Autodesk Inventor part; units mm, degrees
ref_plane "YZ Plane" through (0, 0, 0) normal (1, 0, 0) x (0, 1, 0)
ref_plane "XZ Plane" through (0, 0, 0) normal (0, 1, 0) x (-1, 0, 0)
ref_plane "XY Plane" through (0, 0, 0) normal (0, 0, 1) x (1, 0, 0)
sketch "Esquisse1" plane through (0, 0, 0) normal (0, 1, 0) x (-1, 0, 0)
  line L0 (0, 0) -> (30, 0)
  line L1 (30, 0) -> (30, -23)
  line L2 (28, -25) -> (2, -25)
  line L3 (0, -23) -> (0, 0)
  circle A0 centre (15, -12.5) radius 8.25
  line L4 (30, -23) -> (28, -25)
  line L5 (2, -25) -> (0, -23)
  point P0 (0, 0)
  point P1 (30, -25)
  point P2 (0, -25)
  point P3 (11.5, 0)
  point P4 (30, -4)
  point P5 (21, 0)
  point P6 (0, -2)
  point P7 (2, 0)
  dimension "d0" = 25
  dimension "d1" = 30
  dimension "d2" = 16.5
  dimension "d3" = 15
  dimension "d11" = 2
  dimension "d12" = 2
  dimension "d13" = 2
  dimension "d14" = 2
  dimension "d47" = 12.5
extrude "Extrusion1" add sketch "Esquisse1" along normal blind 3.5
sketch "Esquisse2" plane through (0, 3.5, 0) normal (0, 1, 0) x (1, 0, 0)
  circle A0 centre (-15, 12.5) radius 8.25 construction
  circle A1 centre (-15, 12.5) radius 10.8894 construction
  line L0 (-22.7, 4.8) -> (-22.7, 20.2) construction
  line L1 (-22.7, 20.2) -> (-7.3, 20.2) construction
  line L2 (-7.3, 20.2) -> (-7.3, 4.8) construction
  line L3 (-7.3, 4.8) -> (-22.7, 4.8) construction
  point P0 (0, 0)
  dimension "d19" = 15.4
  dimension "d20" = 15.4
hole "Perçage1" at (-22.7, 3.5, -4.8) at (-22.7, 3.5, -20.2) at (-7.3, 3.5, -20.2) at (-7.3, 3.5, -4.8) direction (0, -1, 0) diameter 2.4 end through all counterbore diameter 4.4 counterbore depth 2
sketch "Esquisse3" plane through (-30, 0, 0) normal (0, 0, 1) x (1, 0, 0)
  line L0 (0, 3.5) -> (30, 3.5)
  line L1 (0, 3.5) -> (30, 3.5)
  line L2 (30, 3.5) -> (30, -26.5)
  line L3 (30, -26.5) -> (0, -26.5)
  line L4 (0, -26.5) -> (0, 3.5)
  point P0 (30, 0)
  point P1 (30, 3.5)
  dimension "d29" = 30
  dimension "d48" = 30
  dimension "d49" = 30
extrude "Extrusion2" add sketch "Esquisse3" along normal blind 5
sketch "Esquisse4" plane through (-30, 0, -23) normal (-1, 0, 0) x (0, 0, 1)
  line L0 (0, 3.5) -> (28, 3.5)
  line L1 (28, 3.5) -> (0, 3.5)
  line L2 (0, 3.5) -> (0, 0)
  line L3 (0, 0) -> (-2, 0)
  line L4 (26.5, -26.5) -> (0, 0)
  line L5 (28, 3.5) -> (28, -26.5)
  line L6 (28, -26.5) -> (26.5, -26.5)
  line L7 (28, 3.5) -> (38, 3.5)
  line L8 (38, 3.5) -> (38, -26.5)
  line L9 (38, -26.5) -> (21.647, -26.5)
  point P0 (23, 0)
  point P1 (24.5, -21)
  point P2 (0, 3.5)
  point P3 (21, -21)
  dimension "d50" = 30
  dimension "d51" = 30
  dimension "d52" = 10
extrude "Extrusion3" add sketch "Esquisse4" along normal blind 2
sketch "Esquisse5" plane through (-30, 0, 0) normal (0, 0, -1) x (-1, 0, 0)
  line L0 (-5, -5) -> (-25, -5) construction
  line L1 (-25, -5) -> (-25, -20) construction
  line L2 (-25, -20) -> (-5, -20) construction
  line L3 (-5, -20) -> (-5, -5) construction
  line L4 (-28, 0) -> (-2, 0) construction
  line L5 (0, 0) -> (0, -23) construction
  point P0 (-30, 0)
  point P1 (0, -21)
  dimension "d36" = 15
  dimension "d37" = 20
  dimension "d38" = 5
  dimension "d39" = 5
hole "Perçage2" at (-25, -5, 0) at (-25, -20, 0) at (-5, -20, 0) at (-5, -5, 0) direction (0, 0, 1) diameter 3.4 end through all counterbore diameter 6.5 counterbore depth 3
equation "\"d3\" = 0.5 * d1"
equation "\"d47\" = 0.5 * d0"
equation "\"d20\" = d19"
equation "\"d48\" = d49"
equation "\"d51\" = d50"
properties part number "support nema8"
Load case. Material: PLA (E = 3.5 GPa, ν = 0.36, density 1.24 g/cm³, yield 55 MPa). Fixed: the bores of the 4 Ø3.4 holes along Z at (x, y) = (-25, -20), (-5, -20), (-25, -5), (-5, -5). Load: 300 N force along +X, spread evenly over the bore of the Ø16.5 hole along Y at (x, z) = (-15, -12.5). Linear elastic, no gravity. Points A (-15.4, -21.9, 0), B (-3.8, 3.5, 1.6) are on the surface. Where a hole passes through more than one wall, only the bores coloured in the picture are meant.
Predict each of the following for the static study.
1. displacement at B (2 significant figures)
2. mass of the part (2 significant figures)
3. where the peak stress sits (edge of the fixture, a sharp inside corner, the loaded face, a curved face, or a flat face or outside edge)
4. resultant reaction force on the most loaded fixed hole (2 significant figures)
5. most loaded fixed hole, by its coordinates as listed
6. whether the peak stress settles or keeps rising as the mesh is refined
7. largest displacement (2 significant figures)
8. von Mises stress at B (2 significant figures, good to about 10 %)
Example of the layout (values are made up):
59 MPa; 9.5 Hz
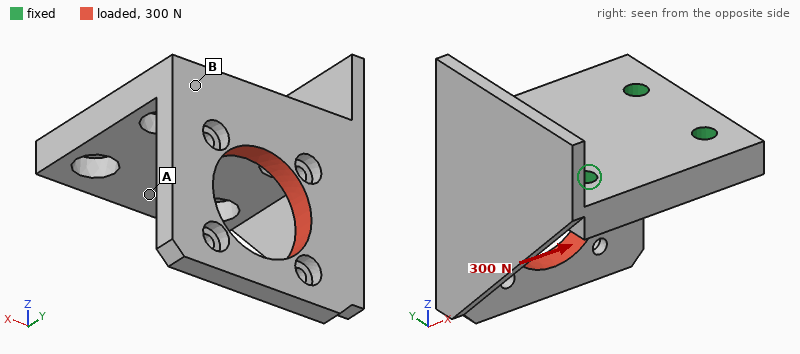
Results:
0.11 mm; 9.1 g; edge of the fixture; 300 N; (-5, -5); keeps rising; 0.44 mm; 9.1 MPa
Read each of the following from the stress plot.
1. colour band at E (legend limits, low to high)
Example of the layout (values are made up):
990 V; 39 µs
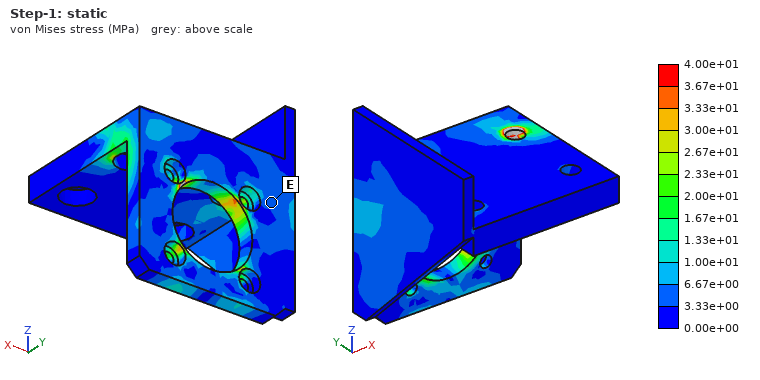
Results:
3.33e+00 to 6.67e+00 MPa
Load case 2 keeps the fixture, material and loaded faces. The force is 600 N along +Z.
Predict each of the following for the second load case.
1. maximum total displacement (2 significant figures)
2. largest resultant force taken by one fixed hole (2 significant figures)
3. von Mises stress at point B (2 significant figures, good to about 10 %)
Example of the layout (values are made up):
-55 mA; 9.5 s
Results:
0.67 mm; 420 N; 9.4 MPa
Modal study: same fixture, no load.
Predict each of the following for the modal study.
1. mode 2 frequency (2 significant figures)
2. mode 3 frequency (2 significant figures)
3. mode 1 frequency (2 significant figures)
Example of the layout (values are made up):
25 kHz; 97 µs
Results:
2700 Hz; 3700 Hz; 1400 Hz
